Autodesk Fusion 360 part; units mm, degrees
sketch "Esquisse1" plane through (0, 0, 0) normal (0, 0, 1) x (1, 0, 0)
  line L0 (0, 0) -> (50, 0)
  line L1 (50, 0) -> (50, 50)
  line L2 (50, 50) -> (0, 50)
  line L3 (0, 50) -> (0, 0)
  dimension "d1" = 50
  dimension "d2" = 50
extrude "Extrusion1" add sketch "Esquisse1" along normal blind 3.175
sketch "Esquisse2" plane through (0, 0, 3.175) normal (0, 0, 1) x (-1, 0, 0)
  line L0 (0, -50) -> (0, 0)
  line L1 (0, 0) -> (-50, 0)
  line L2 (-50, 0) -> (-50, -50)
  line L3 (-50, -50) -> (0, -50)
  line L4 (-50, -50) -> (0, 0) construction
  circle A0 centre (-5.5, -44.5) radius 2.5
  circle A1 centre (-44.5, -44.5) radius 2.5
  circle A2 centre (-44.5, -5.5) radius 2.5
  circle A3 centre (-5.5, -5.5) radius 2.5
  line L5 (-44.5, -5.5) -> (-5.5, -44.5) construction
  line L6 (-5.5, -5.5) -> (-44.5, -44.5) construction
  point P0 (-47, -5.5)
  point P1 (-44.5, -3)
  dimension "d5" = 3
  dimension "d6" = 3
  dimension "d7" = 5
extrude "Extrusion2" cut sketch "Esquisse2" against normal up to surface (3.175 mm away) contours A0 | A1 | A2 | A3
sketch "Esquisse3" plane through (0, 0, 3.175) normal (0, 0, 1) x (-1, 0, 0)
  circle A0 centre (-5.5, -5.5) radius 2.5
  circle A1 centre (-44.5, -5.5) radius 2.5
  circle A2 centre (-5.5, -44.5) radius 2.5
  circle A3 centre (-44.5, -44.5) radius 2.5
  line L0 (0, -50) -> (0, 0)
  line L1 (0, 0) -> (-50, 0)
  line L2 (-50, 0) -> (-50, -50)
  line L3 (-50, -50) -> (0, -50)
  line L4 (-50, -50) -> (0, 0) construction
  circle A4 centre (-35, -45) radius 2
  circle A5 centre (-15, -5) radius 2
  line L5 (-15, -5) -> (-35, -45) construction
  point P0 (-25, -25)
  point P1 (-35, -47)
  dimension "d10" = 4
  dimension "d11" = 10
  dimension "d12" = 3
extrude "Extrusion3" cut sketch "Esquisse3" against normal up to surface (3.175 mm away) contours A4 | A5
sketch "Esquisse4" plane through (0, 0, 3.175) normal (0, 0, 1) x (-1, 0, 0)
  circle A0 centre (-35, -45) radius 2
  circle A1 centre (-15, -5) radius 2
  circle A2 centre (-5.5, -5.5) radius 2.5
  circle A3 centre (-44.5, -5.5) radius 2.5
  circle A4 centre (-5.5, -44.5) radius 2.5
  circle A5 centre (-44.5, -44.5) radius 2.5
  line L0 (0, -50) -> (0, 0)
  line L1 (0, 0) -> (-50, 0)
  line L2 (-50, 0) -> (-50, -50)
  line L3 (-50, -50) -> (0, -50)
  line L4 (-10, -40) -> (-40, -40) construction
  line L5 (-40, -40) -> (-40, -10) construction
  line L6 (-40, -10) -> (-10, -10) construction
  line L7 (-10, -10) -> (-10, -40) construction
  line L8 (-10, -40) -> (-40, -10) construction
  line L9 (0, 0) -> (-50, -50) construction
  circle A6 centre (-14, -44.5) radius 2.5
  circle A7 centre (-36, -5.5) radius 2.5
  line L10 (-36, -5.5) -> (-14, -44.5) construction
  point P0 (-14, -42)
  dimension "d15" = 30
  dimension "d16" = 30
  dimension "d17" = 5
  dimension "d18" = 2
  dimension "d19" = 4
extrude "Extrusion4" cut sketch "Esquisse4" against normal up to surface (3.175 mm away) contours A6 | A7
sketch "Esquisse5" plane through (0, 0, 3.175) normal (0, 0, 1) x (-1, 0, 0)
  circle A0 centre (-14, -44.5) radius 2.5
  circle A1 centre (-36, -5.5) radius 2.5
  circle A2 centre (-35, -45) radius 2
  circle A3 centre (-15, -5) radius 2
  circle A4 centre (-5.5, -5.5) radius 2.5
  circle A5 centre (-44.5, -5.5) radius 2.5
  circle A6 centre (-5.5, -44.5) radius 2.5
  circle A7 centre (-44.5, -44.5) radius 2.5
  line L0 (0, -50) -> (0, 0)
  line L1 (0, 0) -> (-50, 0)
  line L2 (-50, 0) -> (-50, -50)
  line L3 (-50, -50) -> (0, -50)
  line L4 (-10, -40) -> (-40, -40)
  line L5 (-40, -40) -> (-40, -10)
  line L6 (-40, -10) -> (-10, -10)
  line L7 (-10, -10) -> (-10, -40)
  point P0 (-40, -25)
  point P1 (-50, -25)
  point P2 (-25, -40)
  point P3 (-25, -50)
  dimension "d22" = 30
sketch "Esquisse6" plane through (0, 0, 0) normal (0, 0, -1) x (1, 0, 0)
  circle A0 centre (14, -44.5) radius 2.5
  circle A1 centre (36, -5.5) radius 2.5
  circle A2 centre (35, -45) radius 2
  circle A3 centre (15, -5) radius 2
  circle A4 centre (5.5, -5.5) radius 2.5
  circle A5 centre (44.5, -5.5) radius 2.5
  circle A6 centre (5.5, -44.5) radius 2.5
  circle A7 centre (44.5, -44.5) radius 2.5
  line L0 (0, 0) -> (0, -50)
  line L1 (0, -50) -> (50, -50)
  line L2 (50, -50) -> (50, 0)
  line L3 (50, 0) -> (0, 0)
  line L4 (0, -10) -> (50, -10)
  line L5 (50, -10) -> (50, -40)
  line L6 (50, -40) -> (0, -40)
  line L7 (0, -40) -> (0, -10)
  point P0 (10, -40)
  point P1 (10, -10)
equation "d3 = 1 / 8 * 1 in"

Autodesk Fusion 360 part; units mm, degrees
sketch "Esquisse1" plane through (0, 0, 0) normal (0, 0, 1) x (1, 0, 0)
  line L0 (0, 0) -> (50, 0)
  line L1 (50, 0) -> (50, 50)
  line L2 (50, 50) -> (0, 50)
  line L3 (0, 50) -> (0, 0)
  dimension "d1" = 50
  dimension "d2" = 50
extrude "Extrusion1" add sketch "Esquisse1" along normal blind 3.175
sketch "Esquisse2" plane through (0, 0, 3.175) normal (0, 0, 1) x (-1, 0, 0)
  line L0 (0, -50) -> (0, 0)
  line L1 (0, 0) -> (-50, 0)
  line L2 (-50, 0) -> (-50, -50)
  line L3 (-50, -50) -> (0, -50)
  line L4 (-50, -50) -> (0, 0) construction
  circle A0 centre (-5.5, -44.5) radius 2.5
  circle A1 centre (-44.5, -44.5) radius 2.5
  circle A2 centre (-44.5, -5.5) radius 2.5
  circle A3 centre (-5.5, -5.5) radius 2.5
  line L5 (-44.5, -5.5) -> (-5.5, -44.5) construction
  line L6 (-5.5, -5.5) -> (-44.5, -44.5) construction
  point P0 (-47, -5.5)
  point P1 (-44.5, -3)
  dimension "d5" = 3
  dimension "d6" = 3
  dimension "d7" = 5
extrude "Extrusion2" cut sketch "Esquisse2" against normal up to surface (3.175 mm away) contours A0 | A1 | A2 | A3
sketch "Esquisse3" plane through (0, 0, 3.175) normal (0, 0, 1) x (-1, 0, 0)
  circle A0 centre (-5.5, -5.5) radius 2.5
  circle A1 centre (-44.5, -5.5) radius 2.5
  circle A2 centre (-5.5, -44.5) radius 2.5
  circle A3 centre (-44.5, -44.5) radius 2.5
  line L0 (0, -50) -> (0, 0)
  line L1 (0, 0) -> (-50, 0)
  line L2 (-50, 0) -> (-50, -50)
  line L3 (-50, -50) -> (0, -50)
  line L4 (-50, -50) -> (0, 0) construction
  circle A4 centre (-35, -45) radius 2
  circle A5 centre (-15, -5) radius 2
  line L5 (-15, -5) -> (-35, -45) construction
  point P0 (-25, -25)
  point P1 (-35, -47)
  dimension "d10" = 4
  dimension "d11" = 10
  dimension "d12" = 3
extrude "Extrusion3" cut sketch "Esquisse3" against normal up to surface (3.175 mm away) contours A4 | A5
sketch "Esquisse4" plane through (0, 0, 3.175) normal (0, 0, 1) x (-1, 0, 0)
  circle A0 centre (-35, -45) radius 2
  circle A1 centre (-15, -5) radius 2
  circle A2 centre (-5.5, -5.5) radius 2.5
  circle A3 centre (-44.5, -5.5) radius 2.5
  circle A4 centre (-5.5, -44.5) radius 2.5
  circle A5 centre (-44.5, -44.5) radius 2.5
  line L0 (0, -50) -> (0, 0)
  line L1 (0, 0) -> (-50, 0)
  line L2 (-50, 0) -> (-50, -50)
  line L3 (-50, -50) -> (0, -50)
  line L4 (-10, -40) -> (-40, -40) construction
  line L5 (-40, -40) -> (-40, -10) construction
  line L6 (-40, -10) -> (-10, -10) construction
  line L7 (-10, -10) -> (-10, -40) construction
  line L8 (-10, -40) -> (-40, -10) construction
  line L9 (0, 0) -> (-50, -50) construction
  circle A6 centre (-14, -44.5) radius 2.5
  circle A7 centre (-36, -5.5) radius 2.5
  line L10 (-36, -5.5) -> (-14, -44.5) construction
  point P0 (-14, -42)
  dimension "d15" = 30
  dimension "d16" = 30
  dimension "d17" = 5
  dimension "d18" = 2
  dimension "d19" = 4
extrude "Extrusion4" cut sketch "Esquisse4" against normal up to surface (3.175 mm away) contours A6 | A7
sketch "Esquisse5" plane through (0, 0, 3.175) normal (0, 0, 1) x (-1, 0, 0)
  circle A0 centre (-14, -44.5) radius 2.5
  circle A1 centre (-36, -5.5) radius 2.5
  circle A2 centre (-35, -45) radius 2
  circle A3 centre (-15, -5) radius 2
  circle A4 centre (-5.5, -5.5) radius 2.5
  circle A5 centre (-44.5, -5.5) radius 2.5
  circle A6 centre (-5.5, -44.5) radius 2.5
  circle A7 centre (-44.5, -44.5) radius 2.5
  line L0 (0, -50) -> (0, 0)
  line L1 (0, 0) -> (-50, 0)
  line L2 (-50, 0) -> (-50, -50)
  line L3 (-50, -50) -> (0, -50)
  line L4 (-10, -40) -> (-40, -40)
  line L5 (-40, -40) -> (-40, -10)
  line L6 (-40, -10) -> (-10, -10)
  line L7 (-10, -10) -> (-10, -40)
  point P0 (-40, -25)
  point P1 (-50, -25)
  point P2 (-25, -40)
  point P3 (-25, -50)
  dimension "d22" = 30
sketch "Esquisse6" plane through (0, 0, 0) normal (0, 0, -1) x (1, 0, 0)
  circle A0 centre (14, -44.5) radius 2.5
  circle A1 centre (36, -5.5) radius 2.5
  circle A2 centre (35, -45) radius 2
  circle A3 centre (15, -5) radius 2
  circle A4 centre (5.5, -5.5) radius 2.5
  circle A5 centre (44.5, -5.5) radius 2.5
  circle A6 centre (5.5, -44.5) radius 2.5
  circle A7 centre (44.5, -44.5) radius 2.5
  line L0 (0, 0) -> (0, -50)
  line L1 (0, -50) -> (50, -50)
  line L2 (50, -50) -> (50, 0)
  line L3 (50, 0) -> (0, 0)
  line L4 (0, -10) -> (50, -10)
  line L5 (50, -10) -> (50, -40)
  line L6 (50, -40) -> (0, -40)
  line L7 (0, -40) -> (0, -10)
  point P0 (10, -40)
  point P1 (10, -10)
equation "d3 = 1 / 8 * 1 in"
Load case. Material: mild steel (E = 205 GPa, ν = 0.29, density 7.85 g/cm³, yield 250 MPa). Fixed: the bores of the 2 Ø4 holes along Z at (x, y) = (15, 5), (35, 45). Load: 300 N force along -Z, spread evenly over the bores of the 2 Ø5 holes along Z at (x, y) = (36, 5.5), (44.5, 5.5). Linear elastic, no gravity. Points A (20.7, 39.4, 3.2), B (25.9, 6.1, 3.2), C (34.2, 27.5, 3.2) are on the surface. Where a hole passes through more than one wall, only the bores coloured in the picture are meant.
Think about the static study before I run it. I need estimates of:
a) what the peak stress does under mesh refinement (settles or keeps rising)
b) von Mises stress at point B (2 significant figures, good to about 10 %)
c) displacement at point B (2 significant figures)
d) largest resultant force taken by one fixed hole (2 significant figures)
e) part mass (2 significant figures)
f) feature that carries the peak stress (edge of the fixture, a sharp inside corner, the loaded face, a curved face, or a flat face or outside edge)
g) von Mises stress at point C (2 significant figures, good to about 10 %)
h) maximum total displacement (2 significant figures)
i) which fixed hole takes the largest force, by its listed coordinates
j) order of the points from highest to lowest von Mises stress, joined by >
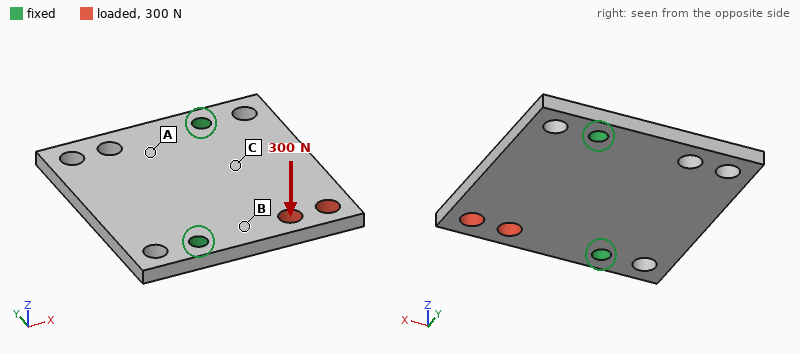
keeps rising
75 MPa
0.022 mm
230 N
59 g
edge of the fixture
44 MPa
0.14 mm
(15, 5)
B > C > A
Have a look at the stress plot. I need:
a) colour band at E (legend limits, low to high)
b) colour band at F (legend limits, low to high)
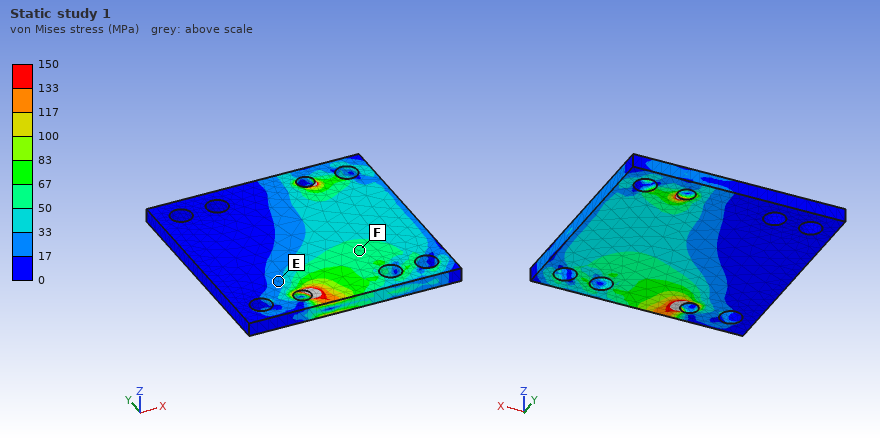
17 to 33 MPa
50 to 67 MPa
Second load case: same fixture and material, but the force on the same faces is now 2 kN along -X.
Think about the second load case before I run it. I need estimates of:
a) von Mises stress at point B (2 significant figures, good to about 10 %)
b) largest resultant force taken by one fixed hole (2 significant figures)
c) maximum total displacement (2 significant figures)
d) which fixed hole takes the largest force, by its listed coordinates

40 MPa
1.9 kN
8.3 µm
(15, 5)
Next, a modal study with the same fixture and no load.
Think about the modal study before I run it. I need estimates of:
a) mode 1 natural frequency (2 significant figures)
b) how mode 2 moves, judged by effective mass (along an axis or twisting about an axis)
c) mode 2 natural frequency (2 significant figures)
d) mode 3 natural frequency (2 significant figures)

2800 Hz
along Z
3700 Hz
8300 Hz
